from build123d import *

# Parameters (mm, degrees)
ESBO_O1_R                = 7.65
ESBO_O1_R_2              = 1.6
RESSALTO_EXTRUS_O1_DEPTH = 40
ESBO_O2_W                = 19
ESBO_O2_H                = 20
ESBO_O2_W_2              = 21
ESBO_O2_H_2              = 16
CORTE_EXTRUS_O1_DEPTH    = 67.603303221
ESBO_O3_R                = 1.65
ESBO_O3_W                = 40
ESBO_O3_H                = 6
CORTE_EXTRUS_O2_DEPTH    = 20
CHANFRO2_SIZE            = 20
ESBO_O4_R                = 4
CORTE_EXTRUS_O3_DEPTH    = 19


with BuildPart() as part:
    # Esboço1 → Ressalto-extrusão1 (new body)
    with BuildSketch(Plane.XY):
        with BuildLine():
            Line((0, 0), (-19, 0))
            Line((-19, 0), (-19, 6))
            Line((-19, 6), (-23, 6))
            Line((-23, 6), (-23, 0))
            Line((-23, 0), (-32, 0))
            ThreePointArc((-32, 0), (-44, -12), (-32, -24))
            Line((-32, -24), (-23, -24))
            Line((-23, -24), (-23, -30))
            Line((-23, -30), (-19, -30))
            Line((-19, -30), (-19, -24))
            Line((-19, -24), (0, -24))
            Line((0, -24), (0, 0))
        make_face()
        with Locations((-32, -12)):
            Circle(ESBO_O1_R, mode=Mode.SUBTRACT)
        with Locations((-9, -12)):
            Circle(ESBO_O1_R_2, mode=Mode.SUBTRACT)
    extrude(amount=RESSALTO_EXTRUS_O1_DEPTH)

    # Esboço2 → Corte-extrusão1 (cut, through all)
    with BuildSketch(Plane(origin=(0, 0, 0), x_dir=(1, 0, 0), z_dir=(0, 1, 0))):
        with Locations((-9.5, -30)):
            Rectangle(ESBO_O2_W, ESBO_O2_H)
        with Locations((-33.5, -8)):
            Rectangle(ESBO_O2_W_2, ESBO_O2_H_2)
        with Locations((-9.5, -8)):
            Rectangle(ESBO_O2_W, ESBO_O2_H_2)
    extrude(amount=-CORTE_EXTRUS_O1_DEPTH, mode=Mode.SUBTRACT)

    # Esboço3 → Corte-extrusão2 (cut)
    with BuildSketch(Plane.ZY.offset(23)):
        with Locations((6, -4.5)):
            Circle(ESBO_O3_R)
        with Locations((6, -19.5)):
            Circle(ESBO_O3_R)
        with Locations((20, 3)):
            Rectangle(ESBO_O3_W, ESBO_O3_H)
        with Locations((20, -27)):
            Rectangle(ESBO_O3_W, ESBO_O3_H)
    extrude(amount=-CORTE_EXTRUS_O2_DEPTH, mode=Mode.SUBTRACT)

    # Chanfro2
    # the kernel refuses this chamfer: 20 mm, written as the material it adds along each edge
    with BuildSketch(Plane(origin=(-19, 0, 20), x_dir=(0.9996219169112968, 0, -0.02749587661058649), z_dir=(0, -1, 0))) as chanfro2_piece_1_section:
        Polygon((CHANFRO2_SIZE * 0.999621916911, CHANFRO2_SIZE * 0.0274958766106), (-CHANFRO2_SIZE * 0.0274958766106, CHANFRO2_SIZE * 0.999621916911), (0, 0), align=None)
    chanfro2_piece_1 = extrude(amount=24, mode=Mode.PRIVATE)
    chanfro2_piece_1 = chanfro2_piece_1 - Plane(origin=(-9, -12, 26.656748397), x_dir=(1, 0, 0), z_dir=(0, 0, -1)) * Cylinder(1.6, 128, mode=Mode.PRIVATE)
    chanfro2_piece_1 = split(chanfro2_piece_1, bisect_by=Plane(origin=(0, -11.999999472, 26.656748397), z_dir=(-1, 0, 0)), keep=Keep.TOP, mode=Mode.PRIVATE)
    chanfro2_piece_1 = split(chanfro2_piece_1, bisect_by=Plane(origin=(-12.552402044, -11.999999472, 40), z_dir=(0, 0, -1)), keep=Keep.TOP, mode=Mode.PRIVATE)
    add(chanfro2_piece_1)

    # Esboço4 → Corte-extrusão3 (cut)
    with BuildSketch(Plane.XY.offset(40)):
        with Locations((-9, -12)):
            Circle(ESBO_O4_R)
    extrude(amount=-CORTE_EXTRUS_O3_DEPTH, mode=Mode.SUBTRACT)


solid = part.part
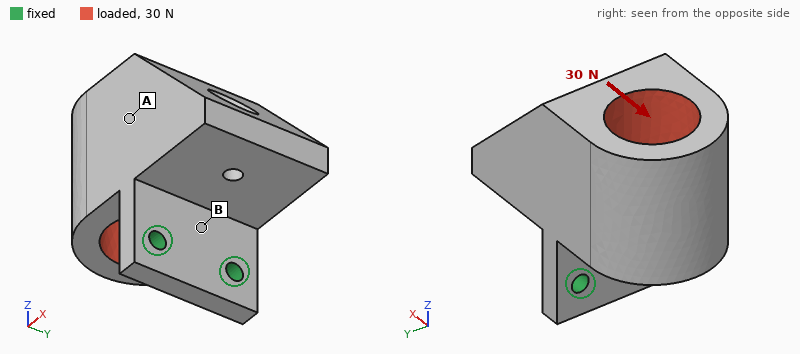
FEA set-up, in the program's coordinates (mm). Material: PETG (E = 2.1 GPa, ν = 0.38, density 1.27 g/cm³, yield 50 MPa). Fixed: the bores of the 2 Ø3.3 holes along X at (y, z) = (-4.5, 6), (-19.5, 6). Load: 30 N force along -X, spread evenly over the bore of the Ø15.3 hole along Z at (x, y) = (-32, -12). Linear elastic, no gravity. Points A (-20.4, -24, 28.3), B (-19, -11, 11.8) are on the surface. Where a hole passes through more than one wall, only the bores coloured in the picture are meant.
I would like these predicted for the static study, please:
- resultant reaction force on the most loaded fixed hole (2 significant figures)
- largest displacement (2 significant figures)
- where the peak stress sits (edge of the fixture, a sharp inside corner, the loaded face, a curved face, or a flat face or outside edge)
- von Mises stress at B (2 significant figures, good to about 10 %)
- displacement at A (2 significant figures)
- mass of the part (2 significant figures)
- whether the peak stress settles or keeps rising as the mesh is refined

15 N
0.71 mm
edge of the fixture
6.0 MPa
0.33 mm
20 g
keeps rising
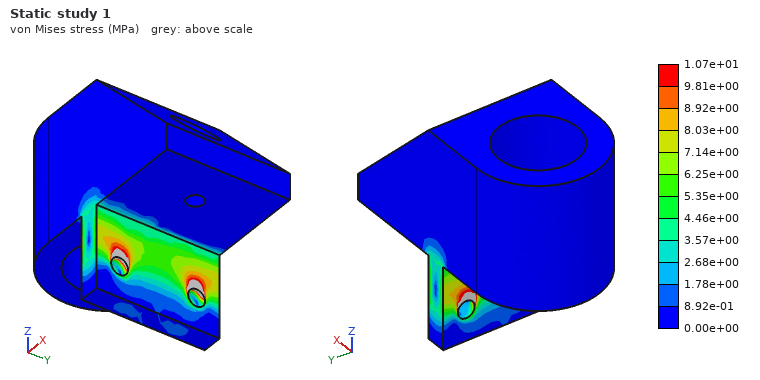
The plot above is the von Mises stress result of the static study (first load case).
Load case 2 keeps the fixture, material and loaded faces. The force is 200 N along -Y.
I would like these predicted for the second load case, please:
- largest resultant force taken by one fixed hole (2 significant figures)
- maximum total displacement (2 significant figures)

300 N
0.67 mm
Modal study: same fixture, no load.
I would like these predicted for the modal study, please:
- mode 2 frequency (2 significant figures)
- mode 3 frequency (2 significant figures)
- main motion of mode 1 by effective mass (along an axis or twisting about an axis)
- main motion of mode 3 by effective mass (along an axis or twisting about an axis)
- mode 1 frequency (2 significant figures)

910 Hz
1500 Hz
along X
along Y
300 Hz
